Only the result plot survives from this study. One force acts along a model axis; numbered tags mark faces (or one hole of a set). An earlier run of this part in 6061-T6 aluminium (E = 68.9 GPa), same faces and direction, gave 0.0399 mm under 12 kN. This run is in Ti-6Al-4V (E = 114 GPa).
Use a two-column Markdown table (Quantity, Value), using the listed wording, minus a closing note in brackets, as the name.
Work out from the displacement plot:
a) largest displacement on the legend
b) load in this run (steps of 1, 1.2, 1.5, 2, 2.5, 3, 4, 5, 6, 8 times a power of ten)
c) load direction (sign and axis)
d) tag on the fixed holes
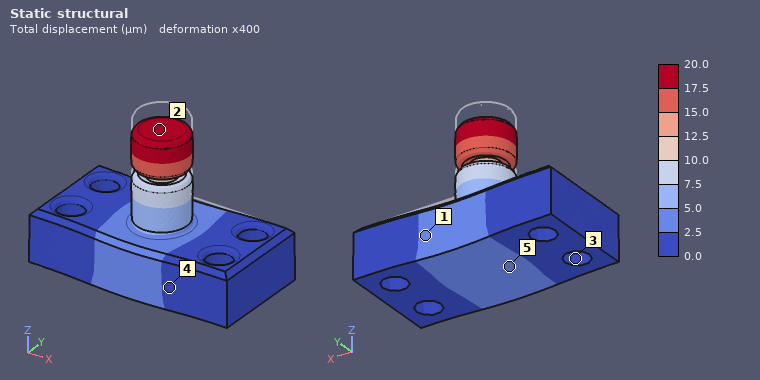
| Quantity | Value |
|---|---|
| largest displacement on the legend | 20.0 µm |
| load in this run | 10 kN |
| load direction | -Z |
| tag on the fixed holes | 3 |
